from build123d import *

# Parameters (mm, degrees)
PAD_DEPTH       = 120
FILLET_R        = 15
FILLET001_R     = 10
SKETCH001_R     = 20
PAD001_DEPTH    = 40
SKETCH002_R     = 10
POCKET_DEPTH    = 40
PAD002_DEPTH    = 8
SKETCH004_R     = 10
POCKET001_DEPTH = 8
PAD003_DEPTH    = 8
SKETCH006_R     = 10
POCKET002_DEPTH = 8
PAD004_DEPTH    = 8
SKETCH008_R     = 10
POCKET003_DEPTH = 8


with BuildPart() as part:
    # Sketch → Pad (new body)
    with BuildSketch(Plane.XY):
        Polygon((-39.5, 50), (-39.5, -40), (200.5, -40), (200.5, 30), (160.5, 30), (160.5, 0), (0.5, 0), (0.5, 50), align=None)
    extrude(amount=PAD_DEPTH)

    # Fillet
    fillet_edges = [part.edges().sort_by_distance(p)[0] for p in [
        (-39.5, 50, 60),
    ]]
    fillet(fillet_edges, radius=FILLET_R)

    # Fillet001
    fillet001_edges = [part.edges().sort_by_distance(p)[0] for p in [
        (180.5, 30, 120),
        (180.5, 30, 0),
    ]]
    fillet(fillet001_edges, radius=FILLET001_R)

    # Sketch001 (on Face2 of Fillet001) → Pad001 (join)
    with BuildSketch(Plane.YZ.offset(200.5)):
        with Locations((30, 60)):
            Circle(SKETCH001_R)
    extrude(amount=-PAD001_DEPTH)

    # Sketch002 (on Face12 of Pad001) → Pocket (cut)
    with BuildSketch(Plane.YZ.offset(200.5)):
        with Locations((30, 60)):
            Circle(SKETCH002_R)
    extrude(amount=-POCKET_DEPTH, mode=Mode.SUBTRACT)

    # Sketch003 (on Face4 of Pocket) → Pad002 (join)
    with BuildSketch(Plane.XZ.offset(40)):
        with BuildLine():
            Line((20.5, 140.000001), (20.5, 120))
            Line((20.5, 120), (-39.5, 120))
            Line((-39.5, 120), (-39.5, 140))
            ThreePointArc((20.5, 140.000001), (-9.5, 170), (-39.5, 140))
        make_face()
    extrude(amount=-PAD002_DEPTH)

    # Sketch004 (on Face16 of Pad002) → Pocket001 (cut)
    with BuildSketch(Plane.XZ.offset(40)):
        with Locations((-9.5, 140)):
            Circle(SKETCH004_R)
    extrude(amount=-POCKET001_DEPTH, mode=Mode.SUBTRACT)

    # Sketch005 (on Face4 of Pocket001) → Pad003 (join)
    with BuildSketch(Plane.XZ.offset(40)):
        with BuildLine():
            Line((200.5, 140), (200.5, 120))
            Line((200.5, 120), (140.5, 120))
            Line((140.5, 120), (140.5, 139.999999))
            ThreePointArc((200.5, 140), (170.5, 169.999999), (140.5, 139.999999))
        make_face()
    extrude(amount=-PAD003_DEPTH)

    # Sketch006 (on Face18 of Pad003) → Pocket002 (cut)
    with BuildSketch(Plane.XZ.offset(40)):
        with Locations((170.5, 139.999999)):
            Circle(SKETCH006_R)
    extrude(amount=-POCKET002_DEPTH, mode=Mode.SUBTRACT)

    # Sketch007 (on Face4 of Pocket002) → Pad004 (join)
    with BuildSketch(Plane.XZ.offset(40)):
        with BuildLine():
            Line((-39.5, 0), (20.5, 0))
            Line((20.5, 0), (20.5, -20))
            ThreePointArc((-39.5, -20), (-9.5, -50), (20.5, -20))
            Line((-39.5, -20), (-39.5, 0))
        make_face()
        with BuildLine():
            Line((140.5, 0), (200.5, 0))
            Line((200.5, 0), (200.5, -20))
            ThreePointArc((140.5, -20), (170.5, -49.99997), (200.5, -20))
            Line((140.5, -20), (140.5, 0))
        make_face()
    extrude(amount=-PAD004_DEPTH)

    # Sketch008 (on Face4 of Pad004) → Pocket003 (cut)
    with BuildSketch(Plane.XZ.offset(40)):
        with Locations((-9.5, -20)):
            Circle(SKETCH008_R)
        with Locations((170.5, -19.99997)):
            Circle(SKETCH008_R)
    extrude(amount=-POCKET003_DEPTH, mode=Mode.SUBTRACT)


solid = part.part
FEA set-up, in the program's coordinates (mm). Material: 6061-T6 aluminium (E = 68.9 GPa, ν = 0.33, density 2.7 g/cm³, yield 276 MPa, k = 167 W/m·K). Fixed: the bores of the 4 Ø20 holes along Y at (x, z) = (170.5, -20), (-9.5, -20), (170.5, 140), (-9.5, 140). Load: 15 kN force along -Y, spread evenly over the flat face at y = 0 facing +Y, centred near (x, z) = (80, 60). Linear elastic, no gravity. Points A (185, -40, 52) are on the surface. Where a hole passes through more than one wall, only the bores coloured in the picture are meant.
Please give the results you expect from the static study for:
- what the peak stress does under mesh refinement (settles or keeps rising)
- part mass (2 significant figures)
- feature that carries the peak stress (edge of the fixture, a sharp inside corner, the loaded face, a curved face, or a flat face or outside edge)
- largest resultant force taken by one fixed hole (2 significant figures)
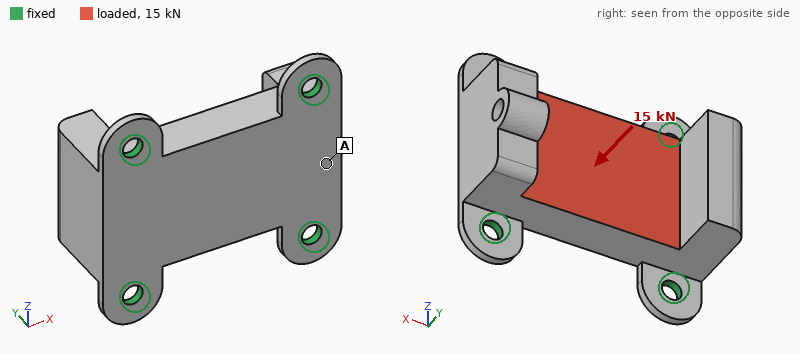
keeps rising
4.4 kg
edge of the fixture
4.7 kN
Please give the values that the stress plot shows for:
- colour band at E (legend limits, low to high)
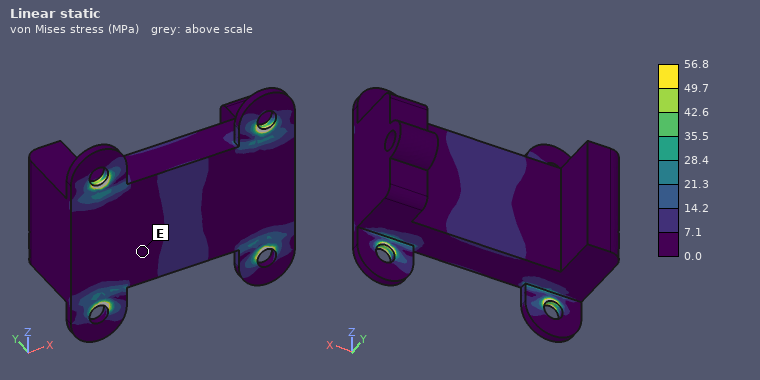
0.0 to 7.1 MPa
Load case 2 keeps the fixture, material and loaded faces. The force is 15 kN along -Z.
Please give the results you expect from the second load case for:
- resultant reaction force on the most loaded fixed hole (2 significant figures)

4.4 kN
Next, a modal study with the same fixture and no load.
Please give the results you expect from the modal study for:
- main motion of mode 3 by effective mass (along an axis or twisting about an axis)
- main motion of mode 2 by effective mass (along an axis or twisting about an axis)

along Z
along X
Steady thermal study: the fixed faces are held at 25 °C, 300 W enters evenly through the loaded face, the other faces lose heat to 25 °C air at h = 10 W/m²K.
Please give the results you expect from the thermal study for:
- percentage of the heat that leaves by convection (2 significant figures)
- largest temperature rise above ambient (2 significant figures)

7.8 %
32 K
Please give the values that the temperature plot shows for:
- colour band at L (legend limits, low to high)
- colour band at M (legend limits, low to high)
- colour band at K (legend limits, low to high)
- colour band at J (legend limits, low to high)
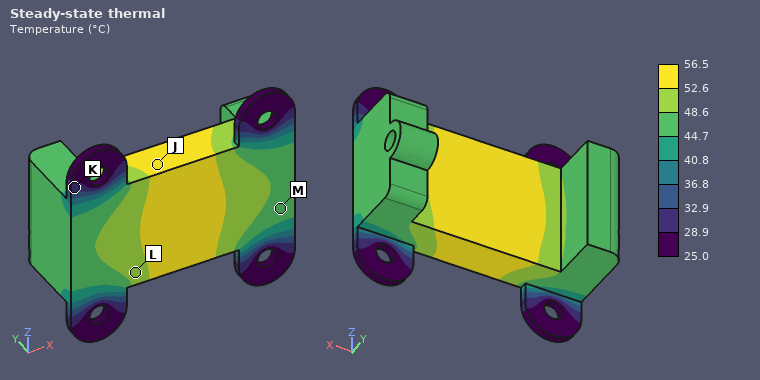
48.6 to 52.6 °C
44.7 to 48.6 °C
28.9 to 32.9 °C
52.6 to 56.5 °C
